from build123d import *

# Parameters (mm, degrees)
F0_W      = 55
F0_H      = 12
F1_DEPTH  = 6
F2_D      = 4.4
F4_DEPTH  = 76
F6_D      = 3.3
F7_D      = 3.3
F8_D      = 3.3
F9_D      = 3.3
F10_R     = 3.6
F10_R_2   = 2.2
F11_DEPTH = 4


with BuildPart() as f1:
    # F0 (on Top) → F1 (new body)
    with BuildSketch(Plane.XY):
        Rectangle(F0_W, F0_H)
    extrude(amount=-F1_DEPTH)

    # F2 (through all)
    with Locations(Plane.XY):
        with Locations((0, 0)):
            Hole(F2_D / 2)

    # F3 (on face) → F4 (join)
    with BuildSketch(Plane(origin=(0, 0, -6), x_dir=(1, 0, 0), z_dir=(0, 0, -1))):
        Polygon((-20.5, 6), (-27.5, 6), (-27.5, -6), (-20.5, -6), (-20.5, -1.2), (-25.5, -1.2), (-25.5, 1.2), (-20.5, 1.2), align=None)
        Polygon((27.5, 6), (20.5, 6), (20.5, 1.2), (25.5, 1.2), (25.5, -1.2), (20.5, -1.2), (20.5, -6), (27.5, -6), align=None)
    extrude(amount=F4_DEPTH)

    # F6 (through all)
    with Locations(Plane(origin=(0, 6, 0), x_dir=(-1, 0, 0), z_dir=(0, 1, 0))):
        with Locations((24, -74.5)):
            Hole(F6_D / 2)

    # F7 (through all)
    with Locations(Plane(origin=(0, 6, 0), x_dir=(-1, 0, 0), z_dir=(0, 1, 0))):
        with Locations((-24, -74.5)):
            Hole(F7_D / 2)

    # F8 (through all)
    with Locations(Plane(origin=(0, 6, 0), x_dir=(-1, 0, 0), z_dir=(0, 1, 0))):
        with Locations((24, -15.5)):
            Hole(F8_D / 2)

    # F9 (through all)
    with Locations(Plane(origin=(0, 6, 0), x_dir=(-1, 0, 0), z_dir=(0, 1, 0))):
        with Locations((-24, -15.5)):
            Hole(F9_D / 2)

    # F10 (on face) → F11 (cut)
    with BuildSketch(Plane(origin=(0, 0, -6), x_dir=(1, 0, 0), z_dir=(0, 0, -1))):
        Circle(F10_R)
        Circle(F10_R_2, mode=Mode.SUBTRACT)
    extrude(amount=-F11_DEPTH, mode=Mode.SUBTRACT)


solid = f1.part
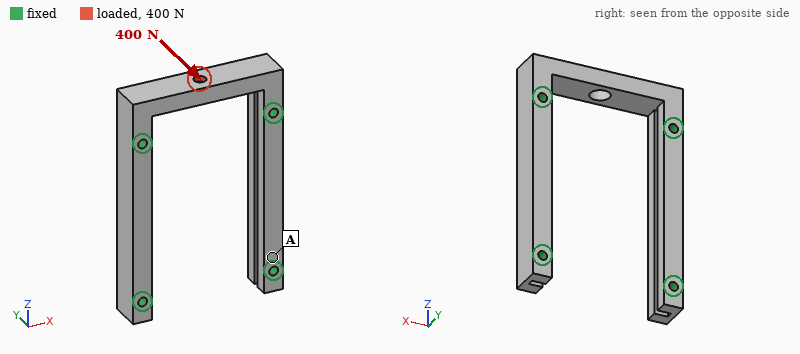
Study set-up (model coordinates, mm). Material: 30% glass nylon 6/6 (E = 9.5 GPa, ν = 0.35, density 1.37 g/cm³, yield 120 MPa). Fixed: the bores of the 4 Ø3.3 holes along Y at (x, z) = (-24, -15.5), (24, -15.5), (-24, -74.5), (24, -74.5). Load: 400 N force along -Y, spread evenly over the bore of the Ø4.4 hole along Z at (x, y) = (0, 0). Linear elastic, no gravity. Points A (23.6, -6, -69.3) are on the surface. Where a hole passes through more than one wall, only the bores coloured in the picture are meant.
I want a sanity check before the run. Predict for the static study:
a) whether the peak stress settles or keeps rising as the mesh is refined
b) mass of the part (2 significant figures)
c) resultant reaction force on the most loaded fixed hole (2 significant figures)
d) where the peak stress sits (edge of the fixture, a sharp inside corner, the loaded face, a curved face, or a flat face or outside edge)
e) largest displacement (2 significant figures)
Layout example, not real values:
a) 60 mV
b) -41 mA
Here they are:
a) keeps rising
b) 20 g
c) 200 N
d) edge of the fixture
e) 0.15 mm
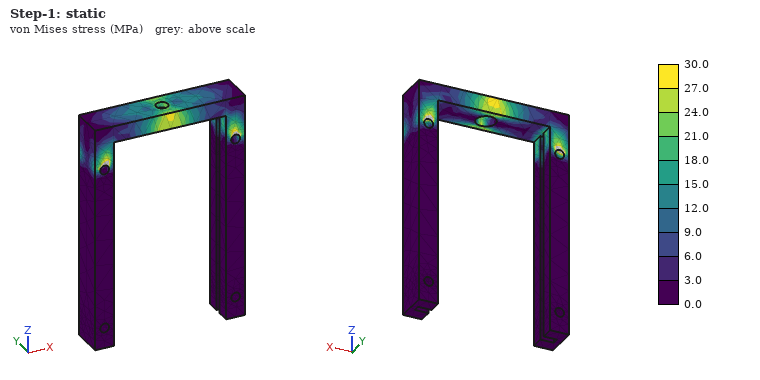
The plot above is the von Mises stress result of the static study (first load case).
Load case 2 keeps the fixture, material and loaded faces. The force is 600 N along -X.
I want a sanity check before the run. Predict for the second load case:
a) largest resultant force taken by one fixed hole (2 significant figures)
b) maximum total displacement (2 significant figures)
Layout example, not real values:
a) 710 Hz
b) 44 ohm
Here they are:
a) 310 N
b) 66 µm
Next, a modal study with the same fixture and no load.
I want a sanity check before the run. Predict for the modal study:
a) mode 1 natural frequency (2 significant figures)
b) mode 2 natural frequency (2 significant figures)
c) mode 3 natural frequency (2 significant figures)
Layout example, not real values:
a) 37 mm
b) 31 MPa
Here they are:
a) 4800 Hz
b) 4900 Hz
c) 5700 Hz
